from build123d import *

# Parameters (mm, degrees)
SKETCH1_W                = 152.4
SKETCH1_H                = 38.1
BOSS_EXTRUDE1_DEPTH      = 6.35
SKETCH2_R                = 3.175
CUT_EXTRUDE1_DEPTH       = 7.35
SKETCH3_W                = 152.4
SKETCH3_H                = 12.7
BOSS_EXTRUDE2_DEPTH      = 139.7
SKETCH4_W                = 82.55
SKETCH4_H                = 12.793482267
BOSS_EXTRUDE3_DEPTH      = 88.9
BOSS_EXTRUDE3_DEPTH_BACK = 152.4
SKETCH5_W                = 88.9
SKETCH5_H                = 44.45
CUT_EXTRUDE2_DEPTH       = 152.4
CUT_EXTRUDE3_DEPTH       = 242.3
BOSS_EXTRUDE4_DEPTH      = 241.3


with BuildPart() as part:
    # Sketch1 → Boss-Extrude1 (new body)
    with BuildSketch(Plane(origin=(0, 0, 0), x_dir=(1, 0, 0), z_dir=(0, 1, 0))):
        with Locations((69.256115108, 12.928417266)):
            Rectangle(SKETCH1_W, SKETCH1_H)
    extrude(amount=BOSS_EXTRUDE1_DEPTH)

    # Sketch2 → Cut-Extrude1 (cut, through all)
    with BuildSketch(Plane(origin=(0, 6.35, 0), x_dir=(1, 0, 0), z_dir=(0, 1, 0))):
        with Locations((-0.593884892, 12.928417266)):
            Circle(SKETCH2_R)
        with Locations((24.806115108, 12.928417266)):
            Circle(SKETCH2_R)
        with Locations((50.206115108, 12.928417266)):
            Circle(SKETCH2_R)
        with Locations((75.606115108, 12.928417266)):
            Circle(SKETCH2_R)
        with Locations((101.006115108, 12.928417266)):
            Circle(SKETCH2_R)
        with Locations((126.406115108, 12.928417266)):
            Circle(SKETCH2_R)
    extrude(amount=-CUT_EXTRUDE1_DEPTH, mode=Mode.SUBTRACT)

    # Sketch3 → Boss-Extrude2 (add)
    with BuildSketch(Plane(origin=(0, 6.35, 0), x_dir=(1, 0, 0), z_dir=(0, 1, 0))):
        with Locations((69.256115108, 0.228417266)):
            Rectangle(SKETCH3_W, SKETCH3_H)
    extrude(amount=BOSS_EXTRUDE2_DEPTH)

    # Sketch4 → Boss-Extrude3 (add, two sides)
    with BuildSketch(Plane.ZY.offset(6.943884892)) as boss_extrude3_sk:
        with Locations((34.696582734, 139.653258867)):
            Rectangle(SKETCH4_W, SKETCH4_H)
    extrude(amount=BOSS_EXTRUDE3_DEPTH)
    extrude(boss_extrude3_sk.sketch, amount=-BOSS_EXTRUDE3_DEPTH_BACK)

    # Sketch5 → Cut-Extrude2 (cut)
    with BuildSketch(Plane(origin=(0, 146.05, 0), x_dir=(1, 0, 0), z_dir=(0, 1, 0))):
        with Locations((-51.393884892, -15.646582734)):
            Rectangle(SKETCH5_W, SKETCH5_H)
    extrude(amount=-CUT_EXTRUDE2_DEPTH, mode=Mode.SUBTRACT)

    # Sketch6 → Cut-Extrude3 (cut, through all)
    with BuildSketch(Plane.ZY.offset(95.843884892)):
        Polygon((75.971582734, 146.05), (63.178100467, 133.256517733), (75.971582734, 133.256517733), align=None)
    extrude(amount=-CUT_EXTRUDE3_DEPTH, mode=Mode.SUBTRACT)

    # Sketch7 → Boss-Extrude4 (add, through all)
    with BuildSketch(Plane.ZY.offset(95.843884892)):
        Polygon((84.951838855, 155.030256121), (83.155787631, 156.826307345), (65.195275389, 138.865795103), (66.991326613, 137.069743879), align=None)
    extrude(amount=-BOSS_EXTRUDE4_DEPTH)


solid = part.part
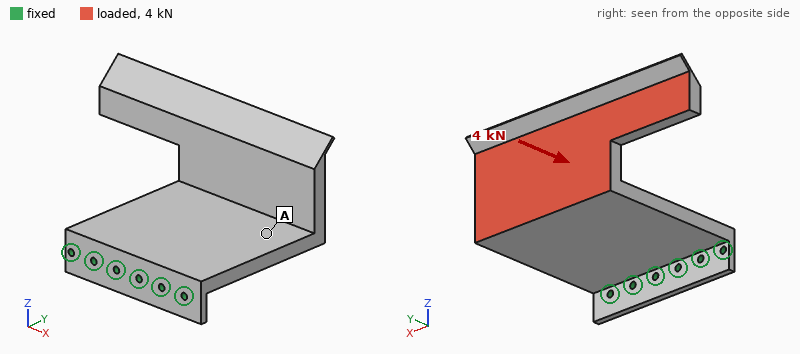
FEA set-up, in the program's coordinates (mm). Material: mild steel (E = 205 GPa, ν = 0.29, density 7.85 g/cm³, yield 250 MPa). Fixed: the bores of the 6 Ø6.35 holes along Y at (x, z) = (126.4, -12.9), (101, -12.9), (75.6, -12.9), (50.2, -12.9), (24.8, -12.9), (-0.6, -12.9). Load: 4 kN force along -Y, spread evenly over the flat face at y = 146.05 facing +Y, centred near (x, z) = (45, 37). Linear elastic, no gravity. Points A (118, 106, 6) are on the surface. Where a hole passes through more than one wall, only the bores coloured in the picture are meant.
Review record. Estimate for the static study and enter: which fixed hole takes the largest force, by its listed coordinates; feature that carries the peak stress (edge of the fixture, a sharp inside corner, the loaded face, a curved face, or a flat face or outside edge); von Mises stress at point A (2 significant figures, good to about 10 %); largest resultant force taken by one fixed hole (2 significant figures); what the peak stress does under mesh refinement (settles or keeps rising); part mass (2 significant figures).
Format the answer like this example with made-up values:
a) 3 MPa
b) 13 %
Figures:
a) (-0.6, -12.9)
b) edge of the fixture
c) 32 MPa
d) 1.4 kN
e) keeps rising
f) 3.7 kg
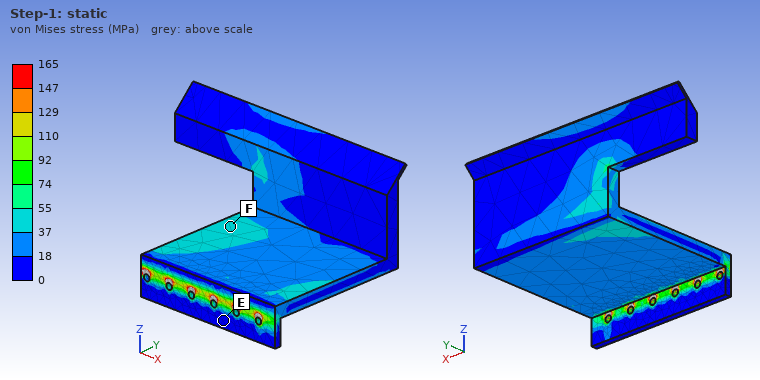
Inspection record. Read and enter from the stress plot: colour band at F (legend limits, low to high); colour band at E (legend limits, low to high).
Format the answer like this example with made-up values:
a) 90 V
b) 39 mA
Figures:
a) 37 to 55 MPa
b) 0 to 18 MPa
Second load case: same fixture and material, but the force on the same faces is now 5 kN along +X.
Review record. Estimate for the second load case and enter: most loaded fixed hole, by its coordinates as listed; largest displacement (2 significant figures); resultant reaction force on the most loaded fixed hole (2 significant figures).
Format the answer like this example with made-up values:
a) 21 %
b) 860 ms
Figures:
a) (126.4, -12.9)
b) 0.38 mm
c) 4.9 kN
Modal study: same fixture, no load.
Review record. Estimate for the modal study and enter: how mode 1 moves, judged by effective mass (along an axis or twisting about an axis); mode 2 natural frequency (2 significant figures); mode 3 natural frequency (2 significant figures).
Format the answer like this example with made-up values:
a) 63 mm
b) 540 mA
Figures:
a) along Z
b) 430 Hz
c) 650 Hz
